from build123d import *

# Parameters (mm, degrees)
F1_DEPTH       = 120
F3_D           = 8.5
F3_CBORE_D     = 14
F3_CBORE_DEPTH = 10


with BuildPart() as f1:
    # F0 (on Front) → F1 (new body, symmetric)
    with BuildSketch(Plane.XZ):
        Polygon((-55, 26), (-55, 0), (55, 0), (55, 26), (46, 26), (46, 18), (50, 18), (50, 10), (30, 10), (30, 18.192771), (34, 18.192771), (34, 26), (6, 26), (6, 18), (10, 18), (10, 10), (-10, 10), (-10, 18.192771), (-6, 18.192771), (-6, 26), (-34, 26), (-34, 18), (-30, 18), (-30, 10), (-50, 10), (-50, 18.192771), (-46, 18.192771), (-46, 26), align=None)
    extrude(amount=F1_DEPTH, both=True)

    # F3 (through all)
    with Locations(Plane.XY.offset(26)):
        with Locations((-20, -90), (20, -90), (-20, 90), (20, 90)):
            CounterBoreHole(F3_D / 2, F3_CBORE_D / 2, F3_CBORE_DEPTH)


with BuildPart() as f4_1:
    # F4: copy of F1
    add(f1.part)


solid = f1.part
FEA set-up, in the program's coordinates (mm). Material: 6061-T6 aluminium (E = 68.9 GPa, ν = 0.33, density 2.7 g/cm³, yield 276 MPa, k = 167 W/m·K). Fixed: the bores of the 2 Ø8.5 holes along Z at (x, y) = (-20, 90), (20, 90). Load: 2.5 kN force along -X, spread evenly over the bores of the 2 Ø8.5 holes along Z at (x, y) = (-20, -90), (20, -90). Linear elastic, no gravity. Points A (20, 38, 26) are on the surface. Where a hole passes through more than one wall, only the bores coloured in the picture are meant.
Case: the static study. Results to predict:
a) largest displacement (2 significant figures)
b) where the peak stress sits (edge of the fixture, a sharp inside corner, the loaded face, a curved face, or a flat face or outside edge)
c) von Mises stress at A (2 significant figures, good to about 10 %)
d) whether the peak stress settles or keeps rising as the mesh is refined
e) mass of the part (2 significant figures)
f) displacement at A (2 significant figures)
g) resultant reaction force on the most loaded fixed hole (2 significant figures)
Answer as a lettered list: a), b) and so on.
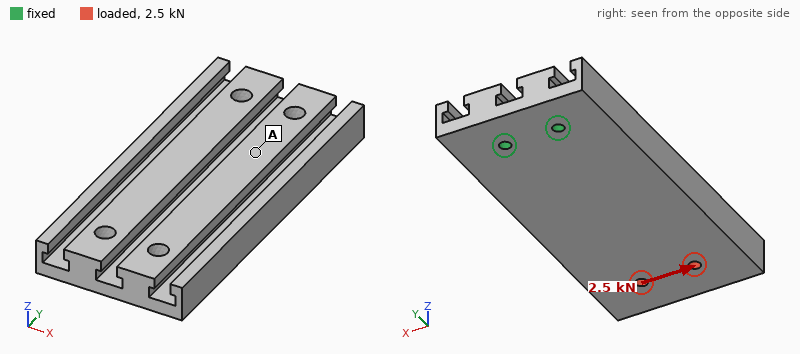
a) 0.13 mm
b) edge of the fixture
c) 4.2 MPa
d) keeps rising
e) 1.3 kg
f) 0.024 mm
g) 9.8 kN
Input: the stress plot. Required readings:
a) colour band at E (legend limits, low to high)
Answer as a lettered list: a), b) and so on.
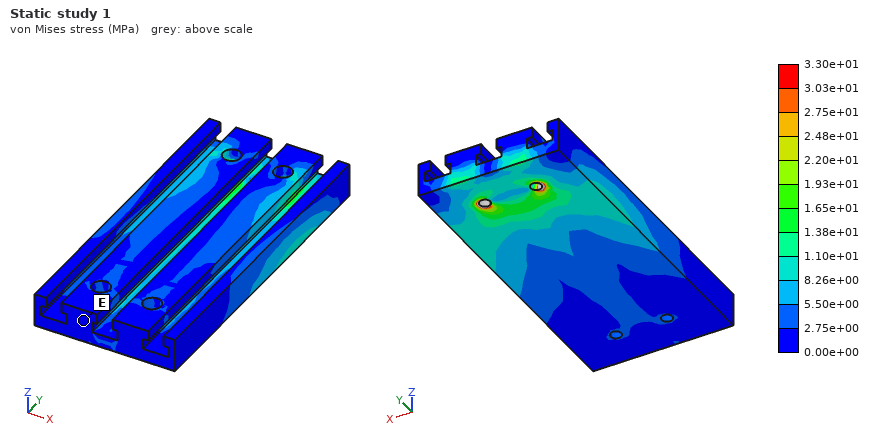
a) 0.00e+00 to 2.75e+00 MPa
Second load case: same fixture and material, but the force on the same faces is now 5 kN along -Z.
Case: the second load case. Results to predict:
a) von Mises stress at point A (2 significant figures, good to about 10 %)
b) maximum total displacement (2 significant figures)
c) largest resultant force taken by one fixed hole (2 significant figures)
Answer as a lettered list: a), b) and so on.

a) 74 MPa
b) 2.2 mm
c) 3.7 kN
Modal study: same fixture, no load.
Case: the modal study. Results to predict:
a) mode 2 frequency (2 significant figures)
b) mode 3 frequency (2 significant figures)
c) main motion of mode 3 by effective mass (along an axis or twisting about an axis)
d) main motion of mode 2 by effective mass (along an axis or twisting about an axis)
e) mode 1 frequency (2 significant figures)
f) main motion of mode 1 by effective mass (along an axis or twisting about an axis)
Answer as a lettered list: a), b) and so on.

a) 920 Hz
b) 1100 Hz
c) along X
d) along X
e) 390 Hz
f) along Z
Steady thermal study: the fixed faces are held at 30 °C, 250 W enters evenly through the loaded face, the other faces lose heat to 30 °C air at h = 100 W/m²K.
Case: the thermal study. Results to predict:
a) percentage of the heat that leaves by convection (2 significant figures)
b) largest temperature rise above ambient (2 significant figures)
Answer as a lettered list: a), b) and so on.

a) 82 %
b) 57 K
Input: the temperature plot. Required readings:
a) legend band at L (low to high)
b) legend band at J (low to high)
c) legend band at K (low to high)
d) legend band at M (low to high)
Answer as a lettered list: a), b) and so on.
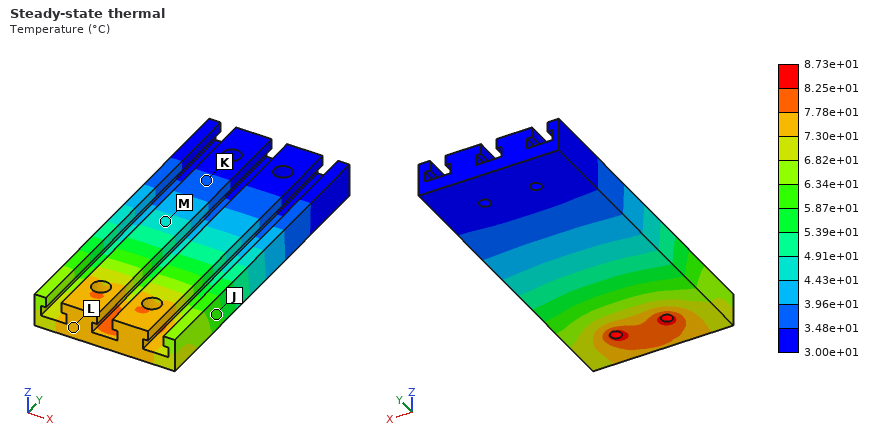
a) 7.30e+01 to 7.78e+01 °C
b) 5.87e+01 to 6.34e+01 °C
c) 3.48e+01 to 3.96e+01 °C
d) 4.43e+01 to 4.91e+01 °C
